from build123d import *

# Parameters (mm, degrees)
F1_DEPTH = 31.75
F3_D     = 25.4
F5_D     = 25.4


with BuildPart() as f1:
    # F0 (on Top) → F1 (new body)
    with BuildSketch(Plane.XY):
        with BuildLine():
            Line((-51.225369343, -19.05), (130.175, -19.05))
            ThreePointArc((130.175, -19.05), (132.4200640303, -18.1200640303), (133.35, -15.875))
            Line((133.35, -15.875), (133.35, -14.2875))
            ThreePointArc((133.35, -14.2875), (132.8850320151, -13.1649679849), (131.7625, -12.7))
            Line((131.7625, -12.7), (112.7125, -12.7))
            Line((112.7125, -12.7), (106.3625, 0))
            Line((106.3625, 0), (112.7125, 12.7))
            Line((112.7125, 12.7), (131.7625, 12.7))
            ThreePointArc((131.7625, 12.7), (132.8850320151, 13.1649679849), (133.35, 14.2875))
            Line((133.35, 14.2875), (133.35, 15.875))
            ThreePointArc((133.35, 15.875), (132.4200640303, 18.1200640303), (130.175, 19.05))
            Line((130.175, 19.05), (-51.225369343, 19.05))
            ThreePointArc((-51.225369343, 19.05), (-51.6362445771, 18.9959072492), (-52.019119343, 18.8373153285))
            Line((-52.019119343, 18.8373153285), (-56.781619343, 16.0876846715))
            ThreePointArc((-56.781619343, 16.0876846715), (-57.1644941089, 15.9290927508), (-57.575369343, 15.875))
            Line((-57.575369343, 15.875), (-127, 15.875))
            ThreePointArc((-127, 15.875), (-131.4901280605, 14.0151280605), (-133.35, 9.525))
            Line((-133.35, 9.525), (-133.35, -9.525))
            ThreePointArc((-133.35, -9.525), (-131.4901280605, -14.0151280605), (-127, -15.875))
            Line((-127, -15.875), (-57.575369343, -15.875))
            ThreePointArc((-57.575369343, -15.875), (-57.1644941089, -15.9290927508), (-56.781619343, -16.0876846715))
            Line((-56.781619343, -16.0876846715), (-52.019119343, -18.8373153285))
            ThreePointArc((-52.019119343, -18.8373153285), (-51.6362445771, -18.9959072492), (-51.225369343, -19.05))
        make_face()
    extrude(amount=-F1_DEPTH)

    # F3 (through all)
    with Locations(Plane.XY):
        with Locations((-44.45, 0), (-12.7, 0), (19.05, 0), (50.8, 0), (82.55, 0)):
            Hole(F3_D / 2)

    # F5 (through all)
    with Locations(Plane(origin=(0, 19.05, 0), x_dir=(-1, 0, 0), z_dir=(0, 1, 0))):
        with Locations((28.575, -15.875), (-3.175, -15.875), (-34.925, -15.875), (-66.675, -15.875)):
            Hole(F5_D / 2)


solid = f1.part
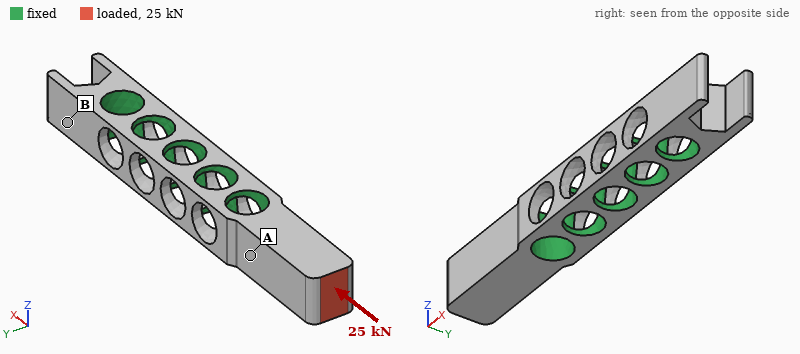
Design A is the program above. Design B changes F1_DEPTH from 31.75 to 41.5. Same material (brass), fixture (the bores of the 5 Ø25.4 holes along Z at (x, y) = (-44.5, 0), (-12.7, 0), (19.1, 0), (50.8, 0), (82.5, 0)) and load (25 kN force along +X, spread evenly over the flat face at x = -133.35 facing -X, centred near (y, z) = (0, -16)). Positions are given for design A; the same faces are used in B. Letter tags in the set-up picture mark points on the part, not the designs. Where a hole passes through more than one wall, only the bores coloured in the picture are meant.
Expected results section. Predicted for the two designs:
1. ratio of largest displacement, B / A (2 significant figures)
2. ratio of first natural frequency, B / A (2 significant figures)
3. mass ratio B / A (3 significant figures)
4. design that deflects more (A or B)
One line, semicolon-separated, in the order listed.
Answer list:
0.77; 1.0; 1.42; A
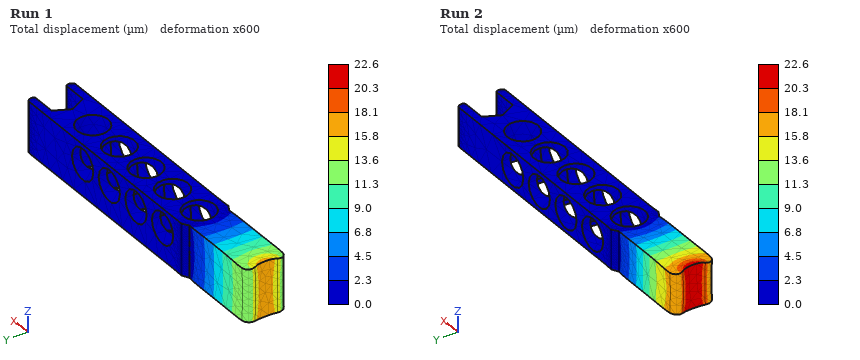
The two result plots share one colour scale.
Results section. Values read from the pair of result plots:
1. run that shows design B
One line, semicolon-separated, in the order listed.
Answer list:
Run 1
